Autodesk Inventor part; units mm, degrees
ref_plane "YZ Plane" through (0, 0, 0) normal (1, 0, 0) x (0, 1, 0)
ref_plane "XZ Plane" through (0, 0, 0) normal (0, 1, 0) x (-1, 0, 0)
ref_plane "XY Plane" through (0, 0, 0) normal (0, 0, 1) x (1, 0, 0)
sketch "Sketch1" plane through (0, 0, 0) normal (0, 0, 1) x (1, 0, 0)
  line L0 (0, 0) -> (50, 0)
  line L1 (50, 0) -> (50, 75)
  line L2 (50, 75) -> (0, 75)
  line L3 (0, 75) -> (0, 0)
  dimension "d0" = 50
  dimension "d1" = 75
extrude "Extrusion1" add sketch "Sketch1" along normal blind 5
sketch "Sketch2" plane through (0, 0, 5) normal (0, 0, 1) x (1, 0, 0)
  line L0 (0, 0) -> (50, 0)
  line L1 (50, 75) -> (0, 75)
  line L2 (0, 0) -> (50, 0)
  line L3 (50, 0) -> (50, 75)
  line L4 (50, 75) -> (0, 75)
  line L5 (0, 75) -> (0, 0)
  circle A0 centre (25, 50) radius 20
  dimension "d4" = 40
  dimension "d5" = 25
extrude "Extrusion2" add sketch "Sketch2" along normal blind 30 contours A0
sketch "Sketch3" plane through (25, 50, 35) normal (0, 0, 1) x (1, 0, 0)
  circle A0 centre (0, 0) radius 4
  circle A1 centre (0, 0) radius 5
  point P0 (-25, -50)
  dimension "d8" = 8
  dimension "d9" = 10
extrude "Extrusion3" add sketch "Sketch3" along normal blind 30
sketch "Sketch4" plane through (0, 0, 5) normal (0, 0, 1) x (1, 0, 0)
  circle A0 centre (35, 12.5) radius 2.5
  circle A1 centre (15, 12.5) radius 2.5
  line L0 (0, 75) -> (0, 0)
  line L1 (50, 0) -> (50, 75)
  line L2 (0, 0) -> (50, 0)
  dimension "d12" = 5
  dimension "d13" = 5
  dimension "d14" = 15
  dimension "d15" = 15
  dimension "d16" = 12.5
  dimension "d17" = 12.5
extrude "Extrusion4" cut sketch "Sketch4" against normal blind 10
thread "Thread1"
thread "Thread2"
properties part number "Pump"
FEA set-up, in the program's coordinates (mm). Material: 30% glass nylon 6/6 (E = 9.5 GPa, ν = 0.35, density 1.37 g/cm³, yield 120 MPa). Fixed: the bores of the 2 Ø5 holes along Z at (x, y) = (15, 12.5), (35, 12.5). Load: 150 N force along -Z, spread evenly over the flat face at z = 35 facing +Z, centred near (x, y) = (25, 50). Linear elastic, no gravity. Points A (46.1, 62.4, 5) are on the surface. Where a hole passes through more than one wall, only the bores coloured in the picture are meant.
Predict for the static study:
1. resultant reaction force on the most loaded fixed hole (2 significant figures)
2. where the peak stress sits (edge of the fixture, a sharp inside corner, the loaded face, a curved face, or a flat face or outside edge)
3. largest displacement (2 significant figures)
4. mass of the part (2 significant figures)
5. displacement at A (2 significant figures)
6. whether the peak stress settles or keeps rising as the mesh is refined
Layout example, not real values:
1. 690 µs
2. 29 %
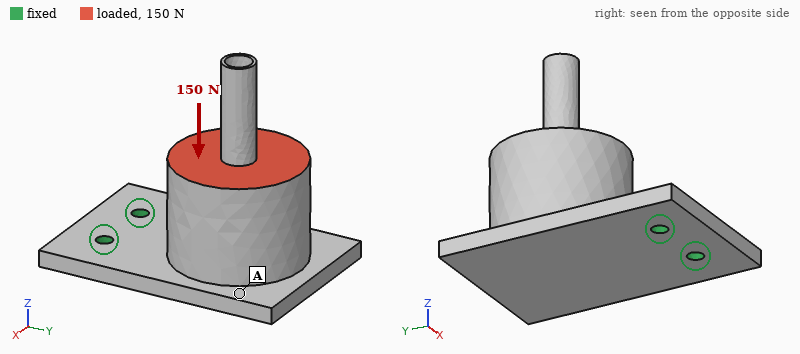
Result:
1. 76 N
2. edge of the fixture
3. 1.2 mm
4. 78 g
5. 0.69 mm
6. keeps rising
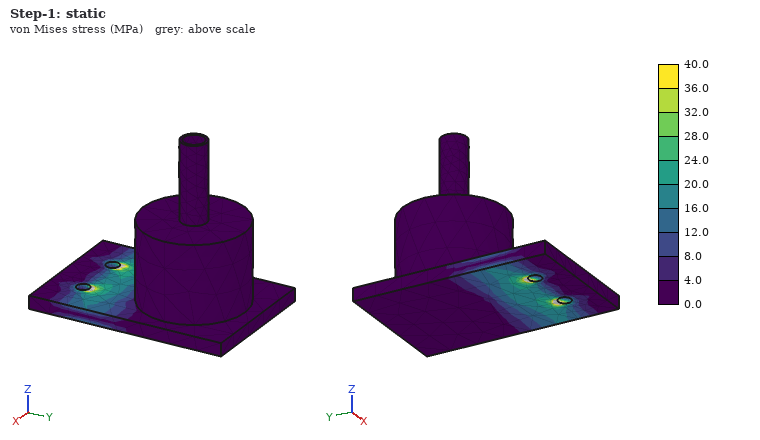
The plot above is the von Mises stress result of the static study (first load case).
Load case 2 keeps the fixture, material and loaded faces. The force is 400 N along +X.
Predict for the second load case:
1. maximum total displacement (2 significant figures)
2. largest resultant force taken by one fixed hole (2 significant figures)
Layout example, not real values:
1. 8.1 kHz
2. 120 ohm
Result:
1. 1.1 mm
2. 820 N
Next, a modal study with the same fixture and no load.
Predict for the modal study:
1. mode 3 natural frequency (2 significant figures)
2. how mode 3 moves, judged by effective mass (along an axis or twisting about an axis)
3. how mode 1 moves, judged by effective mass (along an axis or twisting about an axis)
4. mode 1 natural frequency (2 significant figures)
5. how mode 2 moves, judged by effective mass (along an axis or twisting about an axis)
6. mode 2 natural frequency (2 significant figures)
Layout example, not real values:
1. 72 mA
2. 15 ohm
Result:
1. 2000 Hz
2. along X
3. along Z
4. 270 Hz
5. along X
6. 750 Hz
